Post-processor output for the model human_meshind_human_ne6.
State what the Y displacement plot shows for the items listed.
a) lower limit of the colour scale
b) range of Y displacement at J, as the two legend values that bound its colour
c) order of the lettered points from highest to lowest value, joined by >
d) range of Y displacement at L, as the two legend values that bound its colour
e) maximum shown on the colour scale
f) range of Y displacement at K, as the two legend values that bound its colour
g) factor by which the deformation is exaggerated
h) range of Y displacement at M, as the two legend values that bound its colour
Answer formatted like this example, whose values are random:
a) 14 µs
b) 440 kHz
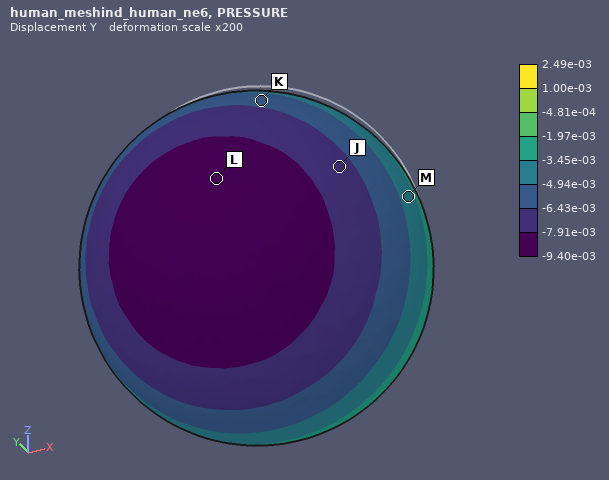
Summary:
a) -9.40e-03
b) -7.91e-03 to -6.43e-03
c) M > K > J > L
d) -9.40e-03 to -7.91e-03
e) 2.49e-03
f) -6.43e-03 to -4.94e-03
g) 200
h) -4.94e-03 to -3.45e-03
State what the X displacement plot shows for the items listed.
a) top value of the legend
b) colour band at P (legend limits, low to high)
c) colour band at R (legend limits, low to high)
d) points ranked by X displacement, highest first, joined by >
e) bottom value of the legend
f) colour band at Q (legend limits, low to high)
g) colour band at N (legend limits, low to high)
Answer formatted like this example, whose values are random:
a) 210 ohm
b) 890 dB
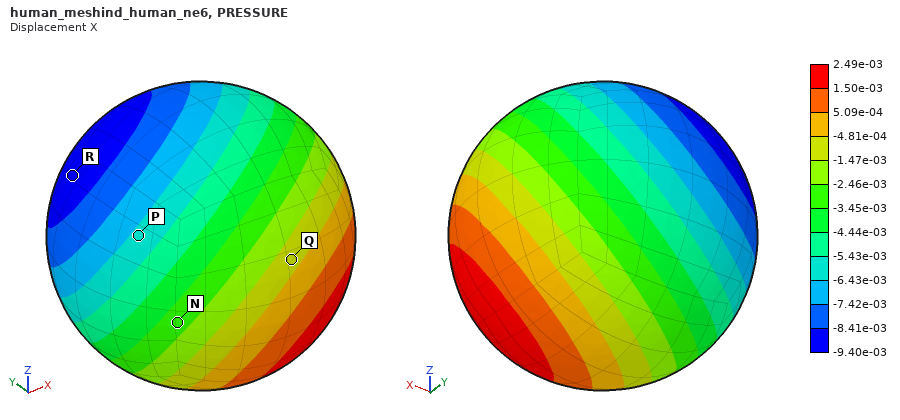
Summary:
a) 2.49e-03
b) -6.43e-03 to -5.43e-03
c) -9.40e-03 to -8.41e-03
d) Q > N > P > R
e) -9.40e-03
f) -1.47e-03 to -4.81e-04
g) -3.45e-03 to -2.46e-03
